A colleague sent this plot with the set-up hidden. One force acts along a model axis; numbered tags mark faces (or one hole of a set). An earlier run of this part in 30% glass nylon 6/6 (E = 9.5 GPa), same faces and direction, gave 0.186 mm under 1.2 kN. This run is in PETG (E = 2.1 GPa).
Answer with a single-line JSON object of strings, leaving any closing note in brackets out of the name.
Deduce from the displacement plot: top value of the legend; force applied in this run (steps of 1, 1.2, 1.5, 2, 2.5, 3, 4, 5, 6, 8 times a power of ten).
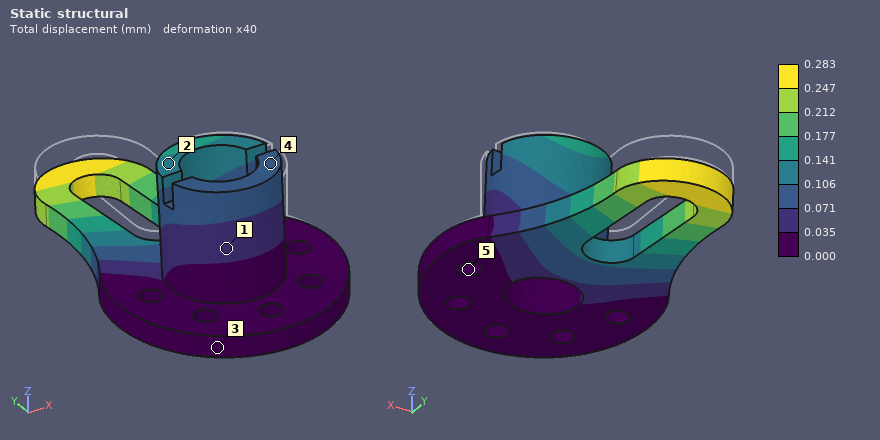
{"top value of the legend": "0.283 mm", "force applied in this run": "400 N"}
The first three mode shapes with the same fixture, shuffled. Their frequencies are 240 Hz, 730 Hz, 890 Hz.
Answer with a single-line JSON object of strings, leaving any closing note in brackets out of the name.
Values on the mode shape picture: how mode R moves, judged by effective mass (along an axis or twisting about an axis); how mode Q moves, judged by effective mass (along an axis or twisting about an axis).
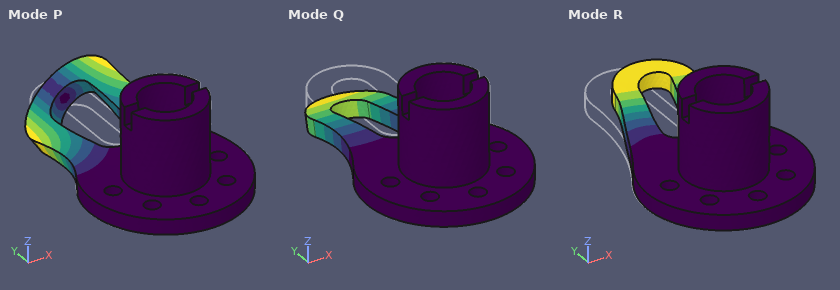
{"how mode R moves, judged by effective mass": "along X", "how mode Q moves, judged by effective mass": "along Z"}
